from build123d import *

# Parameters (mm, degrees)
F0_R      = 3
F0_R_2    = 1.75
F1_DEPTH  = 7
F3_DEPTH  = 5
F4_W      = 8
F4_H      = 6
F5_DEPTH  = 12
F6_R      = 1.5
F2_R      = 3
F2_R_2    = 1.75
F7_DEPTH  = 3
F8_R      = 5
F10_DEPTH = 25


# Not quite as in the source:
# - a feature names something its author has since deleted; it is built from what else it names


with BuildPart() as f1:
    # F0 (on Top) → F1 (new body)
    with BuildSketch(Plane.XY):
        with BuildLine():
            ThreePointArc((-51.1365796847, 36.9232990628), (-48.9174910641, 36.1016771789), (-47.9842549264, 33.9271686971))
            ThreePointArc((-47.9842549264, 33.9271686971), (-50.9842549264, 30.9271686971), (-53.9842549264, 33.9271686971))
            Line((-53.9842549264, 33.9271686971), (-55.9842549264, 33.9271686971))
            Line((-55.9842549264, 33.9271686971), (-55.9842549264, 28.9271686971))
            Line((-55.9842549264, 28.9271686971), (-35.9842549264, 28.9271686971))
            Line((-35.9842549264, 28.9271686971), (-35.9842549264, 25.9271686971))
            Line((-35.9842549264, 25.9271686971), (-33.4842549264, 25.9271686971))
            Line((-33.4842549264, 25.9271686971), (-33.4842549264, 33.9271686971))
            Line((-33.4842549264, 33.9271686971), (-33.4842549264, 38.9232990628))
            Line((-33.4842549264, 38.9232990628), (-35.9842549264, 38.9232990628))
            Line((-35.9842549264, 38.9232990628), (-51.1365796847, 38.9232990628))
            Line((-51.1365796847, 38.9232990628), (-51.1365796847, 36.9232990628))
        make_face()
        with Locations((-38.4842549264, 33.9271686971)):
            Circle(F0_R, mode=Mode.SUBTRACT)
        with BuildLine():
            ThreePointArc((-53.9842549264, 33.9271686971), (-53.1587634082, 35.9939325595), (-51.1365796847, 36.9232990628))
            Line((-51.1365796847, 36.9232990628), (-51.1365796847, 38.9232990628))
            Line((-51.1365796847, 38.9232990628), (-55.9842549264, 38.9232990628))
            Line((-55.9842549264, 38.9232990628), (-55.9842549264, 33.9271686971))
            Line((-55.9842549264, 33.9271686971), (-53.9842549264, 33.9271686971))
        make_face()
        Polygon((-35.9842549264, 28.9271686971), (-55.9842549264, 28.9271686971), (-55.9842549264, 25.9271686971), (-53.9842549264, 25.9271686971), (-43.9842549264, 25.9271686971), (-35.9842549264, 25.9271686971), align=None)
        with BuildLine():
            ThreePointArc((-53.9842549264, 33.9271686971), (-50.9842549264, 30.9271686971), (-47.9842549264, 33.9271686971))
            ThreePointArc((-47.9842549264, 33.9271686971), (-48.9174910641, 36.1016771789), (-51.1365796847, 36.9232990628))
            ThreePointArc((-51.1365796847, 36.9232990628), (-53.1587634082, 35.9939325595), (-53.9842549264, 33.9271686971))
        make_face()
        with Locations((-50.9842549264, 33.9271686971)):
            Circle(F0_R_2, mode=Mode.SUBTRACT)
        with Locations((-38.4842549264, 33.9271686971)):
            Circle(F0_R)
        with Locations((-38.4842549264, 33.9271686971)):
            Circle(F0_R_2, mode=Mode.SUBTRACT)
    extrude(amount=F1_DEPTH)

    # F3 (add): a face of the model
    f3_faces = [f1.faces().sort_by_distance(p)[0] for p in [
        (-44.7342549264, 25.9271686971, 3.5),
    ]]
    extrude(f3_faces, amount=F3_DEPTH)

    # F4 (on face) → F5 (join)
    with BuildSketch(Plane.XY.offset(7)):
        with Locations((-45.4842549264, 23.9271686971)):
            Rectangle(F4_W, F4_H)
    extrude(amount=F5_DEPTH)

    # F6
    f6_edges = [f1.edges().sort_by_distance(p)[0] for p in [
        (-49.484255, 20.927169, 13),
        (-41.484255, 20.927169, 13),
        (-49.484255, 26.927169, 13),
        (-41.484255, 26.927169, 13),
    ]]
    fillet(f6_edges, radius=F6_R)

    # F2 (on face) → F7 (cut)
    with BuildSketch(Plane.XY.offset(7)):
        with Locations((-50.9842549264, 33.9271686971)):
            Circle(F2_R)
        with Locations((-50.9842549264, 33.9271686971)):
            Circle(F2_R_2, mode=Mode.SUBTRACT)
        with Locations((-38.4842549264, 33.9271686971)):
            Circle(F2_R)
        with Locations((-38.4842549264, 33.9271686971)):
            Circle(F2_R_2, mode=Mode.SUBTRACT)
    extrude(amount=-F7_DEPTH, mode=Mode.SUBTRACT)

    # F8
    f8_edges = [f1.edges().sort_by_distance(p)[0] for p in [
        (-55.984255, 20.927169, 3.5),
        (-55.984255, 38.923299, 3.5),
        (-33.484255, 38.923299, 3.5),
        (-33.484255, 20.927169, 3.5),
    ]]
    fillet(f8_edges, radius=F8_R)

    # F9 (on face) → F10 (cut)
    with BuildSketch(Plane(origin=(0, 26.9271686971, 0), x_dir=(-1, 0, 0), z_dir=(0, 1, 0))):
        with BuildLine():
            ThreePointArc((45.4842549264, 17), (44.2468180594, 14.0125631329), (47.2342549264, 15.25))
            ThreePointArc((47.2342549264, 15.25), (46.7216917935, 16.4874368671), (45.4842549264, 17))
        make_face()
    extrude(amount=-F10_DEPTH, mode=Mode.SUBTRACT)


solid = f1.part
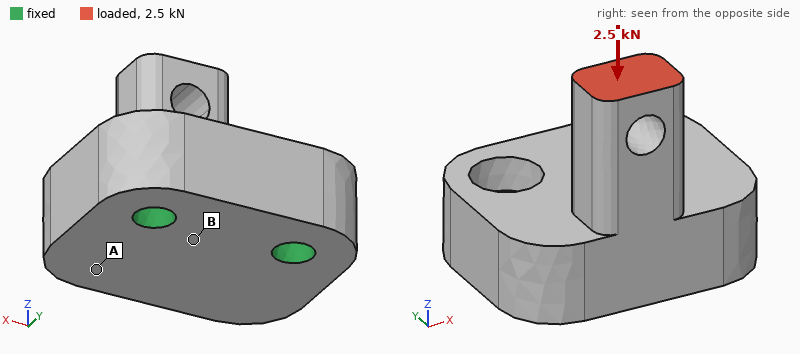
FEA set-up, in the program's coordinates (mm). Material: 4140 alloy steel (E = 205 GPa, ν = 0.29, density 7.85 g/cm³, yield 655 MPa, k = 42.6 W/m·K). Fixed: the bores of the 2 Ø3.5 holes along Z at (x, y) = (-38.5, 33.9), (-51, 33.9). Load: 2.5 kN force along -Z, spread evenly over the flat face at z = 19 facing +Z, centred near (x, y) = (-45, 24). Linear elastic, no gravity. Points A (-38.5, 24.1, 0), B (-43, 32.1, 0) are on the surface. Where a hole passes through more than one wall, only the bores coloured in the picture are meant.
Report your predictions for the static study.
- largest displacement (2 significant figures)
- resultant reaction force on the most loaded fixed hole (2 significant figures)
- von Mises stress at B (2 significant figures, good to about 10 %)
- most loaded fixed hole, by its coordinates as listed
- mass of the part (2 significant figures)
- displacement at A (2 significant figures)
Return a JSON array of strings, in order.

["50 µm", "1.4 kN", "96 MPa", "(-51, 33.9)", "23 g", "18 µm"]
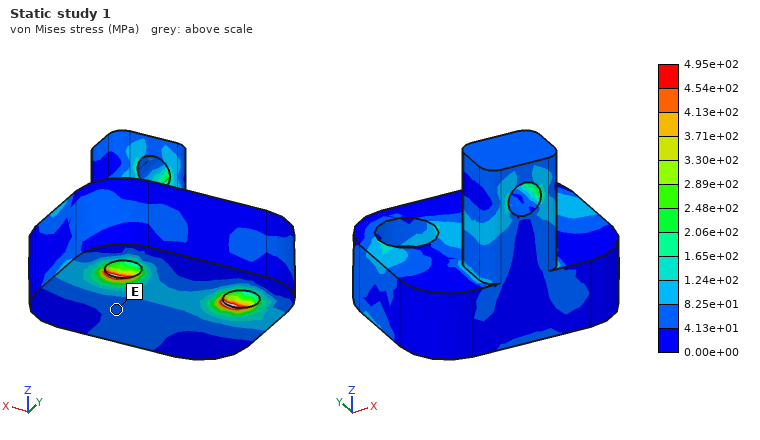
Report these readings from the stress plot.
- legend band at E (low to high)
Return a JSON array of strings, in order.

["4.13e+01 to 8.25e+01 MPa"]
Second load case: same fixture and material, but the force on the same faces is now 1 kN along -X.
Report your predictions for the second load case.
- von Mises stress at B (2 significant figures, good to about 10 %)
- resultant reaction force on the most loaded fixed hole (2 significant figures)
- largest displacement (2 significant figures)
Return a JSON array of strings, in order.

["33 MPa", "1.5 kN", "43 µm"]
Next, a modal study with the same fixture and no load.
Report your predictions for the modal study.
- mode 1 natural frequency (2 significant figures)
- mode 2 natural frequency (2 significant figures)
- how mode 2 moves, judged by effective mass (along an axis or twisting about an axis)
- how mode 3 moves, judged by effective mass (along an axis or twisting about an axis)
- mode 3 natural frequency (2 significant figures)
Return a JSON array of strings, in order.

["12 kHz", "21 kHz", "along X", "along Z", "28 kHz"]
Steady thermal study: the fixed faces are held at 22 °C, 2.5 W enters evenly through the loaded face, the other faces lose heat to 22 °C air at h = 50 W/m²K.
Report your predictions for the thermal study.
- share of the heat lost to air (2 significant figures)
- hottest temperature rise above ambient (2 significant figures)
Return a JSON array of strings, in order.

["15 %", "24 K"]
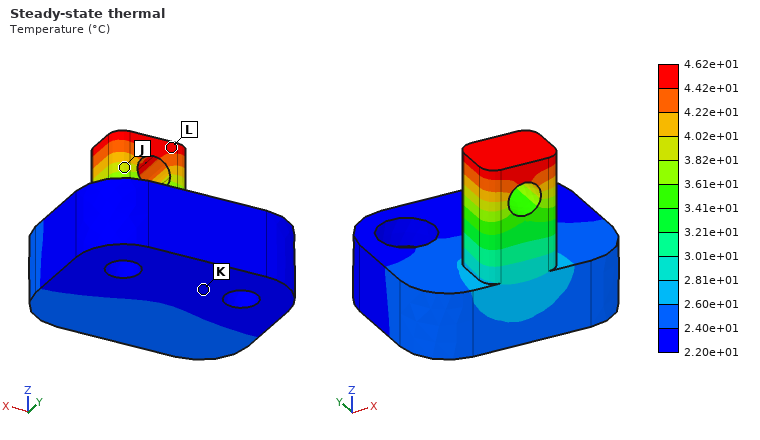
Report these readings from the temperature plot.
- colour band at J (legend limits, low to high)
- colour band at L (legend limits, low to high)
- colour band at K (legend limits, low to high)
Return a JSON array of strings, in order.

["3.82e+01 to 4.02e+01 °C", "4.42e+01 to 4.62e+01 °C", "2.20e+01 to 2.40e+01 °C"]
